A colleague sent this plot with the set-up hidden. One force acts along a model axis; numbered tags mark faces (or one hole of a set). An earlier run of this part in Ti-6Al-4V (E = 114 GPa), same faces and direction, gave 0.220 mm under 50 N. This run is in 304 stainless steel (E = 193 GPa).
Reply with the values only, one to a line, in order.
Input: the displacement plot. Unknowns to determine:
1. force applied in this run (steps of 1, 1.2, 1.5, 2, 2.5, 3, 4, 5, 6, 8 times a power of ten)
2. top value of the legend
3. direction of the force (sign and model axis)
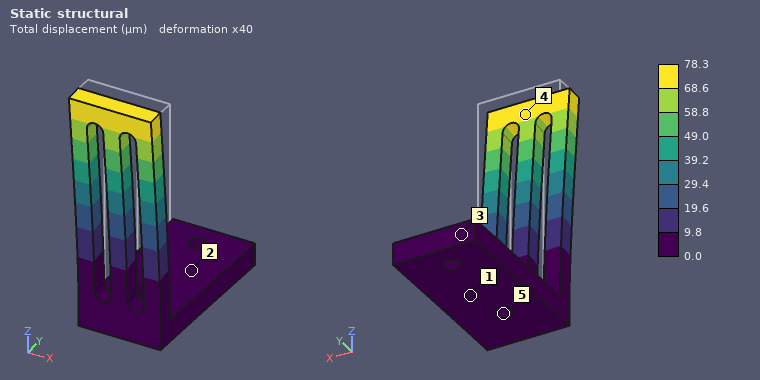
30 N
78.3 µm
-Y
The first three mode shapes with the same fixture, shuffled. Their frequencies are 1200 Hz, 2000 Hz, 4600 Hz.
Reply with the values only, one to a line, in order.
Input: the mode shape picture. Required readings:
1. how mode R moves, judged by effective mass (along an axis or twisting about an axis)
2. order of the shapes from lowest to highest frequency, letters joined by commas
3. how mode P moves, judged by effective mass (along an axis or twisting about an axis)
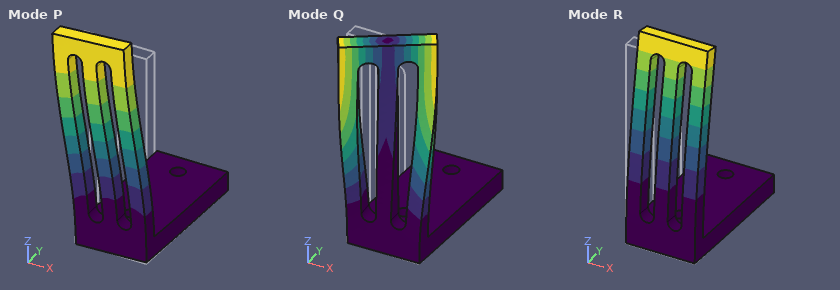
along Y
R, P, Q
along X
